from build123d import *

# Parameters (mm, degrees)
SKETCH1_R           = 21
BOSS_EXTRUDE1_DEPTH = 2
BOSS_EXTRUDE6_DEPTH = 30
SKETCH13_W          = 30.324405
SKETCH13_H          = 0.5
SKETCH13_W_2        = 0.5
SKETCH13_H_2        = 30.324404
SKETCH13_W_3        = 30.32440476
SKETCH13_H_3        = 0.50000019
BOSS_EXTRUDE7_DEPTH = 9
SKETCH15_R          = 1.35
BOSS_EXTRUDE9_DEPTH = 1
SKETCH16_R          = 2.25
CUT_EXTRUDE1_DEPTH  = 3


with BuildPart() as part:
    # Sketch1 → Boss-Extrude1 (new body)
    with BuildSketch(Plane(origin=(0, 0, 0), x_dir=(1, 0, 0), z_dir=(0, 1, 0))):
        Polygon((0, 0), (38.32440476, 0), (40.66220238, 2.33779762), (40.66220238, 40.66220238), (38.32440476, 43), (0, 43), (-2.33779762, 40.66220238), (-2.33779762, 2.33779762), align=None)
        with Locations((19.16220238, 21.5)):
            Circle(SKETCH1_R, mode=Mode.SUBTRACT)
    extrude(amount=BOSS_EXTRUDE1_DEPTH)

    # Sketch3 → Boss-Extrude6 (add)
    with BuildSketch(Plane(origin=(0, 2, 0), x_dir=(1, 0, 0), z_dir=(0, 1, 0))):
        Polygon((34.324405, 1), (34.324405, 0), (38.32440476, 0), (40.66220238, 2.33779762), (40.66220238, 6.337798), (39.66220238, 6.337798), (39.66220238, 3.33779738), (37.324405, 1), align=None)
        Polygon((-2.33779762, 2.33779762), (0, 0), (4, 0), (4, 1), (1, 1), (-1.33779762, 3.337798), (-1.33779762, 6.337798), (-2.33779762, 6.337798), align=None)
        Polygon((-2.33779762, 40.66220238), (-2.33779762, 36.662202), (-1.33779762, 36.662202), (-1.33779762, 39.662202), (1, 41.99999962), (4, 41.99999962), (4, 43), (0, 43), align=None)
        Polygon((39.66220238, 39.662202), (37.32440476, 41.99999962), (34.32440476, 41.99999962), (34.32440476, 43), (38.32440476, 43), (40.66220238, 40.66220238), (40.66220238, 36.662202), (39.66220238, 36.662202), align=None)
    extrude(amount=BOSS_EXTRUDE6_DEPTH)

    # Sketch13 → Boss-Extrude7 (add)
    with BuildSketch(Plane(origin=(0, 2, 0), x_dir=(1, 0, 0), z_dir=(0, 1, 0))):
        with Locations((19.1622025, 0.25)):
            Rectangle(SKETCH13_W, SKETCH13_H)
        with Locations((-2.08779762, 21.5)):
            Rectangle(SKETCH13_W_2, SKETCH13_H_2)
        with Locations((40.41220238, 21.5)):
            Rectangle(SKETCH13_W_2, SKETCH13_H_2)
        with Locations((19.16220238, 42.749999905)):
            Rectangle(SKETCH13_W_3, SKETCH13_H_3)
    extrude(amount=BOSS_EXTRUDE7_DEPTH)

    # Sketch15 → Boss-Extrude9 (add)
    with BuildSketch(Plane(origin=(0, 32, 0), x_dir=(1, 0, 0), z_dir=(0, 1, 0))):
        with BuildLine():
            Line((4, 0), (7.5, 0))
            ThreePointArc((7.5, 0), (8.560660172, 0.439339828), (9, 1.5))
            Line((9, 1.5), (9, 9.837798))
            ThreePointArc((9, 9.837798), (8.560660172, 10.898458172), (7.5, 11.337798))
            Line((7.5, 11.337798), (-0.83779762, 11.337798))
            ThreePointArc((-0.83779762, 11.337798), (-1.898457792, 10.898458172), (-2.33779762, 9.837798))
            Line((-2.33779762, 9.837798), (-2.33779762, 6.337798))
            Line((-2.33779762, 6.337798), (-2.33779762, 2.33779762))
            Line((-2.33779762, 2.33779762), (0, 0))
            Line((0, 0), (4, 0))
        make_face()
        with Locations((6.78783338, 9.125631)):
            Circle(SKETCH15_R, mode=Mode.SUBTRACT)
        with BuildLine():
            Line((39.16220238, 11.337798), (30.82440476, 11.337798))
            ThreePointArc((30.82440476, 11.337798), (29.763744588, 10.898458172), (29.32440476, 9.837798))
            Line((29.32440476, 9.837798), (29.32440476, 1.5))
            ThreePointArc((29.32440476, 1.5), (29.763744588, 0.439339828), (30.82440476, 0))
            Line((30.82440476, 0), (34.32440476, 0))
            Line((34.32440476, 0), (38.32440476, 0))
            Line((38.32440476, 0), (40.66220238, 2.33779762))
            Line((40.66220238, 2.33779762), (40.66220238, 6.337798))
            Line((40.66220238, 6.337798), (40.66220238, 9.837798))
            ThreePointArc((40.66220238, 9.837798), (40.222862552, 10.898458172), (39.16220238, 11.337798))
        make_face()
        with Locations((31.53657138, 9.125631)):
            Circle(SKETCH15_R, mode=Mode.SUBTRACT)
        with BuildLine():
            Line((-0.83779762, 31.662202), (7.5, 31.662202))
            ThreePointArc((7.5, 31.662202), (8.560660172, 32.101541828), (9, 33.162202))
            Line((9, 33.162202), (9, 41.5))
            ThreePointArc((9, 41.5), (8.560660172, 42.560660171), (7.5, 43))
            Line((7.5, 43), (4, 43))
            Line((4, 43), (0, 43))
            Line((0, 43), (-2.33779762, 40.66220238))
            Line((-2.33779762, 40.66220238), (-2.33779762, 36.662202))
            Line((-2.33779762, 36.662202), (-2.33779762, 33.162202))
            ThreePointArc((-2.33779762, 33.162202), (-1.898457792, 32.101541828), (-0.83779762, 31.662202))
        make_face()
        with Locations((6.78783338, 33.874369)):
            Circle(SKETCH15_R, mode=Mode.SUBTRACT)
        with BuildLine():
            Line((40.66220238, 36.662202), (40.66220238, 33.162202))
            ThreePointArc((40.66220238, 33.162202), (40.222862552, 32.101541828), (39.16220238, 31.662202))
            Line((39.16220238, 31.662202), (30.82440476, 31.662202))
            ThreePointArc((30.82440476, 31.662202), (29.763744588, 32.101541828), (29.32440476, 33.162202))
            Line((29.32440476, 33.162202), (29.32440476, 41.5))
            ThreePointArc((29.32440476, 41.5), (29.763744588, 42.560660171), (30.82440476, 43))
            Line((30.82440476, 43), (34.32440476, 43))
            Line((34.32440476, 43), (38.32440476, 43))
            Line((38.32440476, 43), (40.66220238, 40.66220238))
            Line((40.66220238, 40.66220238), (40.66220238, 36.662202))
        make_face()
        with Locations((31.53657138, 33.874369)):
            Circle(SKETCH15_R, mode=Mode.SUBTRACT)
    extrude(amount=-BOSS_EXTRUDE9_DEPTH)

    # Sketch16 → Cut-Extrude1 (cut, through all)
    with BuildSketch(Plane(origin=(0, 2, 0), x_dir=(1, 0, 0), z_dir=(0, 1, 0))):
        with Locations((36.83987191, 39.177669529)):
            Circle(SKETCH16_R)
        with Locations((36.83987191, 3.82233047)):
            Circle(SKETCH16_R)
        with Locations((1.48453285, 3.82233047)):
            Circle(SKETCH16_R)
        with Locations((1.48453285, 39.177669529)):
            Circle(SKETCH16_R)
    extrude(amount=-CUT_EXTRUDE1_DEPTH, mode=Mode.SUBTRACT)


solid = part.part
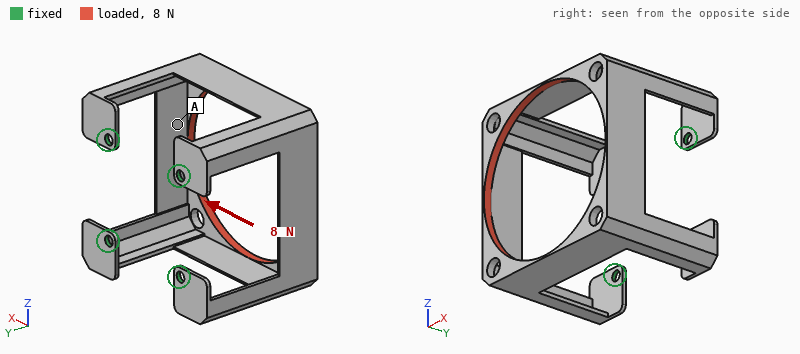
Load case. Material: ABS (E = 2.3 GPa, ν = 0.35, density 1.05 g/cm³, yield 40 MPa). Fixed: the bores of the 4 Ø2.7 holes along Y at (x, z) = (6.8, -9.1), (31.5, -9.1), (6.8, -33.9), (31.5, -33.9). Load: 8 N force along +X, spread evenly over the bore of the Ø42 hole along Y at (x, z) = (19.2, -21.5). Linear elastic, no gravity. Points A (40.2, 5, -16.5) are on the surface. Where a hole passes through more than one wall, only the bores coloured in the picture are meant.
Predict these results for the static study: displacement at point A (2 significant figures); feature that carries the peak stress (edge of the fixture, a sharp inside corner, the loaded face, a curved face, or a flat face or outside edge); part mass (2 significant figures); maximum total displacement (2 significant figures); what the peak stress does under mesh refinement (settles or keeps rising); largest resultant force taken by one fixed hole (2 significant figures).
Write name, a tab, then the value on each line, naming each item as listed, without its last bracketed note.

displacement at point A	0.68 mm
feature that carries the peak stress	edge of the fixture
part mass	3.3 g
maximum total displacement	0.79 mm
what the peak stress does under mesh refinement	keeps rising
largest resultant force taken by one fixed hole	4.1 N
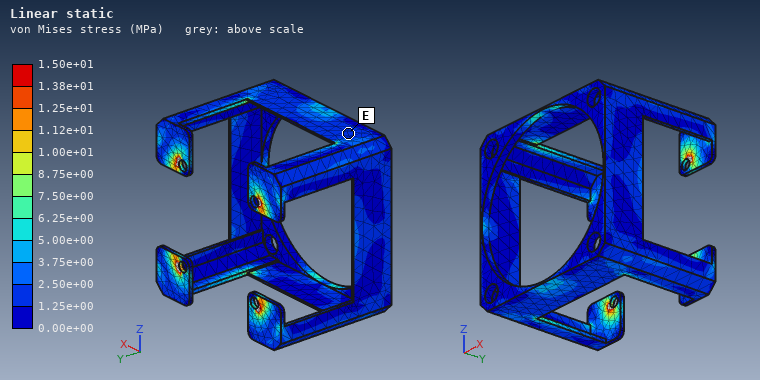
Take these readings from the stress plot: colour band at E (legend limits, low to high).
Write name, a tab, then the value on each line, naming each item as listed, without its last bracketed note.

colour band at E	1.25e+00 to 2.50e+00 MPa
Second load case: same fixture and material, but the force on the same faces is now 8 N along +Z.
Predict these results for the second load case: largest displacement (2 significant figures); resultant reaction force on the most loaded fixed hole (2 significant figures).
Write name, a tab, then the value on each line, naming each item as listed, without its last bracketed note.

largest displacement	0.79 mm
resultant reaction force on the most loaded fixed hole	4.1 N
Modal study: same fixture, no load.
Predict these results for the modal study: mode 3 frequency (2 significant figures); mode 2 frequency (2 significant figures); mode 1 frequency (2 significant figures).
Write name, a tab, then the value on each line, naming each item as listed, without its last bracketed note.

mode 3 frequency	400 Hz
mode 2 frequency	390 Hz
mode 1 frequency	390 Hz
